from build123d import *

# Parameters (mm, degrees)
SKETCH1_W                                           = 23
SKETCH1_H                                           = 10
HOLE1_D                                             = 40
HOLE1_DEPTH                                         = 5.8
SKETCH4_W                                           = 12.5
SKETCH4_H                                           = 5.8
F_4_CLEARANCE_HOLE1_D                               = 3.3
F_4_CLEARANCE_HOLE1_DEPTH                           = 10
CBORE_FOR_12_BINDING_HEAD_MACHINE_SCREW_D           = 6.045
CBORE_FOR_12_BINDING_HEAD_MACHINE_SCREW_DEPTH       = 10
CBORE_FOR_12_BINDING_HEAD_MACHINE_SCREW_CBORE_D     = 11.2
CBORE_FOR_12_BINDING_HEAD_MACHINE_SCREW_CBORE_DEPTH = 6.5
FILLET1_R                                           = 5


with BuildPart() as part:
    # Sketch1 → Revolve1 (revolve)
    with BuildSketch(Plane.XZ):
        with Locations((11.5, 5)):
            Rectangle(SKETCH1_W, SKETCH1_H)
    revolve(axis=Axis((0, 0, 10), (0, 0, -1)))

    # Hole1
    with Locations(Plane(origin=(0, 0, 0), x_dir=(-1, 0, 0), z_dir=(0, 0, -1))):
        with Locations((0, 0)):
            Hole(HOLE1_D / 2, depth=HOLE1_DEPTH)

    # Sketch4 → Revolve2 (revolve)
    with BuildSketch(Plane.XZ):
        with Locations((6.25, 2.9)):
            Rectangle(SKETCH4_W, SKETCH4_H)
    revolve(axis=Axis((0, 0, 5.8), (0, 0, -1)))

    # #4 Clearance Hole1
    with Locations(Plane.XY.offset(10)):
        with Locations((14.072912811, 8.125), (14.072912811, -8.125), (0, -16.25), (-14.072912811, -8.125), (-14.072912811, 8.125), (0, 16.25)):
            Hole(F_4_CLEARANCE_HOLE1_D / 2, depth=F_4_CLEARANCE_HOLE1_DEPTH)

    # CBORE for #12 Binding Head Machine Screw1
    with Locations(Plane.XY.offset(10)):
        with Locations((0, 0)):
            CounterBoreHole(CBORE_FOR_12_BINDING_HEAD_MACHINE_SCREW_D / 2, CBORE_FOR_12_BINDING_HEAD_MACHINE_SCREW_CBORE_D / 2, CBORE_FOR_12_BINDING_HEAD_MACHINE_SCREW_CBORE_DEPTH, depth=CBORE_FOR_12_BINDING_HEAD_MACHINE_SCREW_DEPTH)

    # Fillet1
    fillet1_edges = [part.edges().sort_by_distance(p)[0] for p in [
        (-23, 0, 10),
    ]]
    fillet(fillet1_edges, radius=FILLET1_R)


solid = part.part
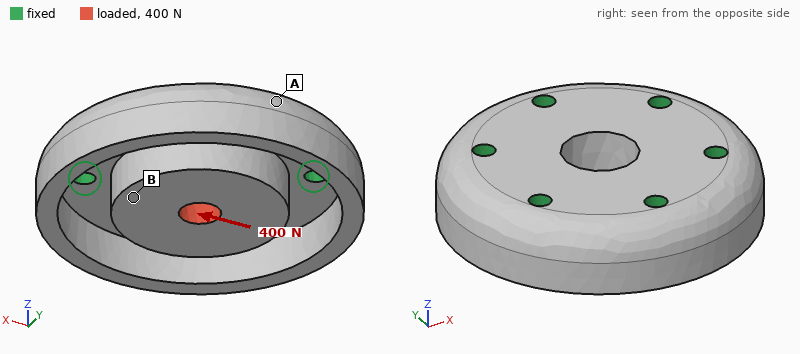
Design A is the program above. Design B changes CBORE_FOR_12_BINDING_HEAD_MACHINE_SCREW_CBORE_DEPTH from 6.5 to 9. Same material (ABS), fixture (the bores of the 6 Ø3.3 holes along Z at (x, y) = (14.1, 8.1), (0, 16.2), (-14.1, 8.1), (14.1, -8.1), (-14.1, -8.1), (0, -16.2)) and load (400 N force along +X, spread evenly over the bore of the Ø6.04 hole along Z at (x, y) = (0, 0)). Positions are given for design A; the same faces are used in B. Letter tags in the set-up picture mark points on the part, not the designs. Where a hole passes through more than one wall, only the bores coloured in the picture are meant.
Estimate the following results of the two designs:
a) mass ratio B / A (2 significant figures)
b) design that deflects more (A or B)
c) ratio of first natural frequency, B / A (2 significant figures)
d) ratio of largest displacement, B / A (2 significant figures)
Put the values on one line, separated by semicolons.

0.98; B; 1.00; 2.1
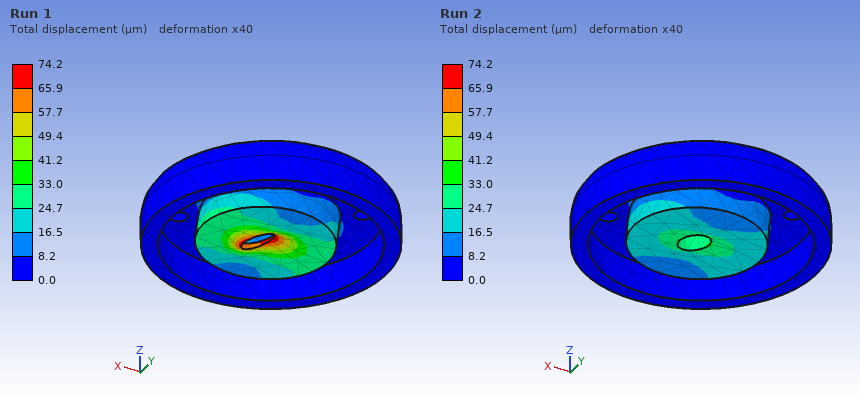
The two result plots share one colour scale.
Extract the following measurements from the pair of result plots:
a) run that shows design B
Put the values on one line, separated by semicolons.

Run 1
